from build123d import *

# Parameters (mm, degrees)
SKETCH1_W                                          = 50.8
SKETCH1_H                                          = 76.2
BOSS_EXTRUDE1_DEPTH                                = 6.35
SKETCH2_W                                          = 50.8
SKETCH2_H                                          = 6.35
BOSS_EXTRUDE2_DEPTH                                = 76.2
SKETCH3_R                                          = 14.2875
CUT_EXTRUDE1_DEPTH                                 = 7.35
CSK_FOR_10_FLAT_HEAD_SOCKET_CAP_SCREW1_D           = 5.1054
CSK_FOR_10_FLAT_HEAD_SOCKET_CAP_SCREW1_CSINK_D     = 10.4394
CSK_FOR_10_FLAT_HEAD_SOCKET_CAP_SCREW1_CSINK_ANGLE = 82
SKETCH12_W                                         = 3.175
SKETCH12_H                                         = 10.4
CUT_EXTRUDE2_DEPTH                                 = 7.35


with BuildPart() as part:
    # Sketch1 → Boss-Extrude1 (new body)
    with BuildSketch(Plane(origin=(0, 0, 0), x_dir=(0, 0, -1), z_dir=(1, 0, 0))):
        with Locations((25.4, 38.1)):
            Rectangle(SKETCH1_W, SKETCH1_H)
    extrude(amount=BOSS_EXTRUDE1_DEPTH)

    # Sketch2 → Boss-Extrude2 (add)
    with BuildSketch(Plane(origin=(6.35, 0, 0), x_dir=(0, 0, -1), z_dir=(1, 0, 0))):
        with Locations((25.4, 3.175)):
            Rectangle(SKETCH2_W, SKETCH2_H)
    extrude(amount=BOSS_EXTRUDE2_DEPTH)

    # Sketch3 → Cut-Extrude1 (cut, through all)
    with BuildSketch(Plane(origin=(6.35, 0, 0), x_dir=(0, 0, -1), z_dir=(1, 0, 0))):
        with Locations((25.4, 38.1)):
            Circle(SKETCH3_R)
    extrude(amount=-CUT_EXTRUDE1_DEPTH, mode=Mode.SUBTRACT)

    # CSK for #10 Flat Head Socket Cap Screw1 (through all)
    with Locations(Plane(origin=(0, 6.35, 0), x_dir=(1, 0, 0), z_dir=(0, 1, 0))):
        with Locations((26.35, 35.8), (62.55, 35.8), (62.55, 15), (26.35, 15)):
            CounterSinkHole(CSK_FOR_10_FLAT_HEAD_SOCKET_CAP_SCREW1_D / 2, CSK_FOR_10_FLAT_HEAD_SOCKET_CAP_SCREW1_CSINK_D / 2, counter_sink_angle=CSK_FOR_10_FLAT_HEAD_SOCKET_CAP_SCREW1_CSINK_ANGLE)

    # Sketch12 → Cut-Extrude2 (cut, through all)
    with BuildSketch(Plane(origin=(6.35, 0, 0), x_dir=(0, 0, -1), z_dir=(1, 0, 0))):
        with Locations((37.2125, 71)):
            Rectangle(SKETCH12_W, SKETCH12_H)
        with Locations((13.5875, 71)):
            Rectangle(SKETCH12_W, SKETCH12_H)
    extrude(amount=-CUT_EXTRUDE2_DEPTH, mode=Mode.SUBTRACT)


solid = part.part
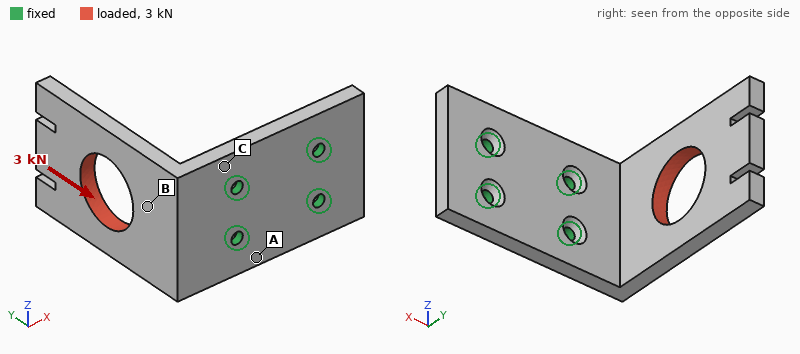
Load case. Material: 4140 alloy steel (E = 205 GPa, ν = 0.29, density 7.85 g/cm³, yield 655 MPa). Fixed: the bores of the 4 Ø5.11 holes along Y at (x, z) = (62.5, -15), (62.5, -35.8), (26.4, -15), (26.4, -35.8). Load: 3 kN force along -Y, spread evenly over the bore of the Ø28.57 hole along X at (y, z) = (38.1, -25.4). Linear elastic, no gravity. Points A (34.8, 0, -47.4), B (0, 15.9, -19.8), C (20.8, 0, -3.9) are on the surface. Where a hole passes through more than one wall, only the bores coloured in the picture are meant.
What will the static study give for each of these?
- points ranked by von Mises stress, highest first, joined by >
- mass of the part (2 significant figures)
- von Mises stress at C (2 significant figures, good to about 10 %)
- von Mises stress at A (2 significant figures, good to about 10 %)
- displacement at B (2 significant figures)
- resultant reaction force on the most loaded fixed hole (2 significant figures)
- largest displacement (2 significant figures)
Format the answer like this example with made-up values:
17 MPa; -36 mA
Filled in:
C > A > B; 340 g; 130 MPa; 54 MPa; 0.12 mm; 2.4 kN; 0.38 mm
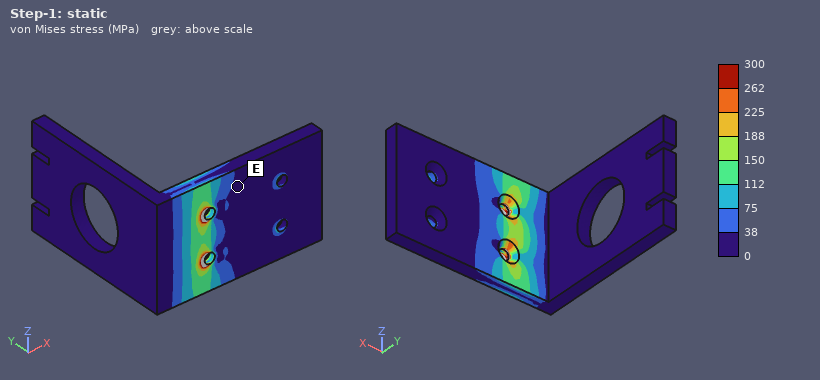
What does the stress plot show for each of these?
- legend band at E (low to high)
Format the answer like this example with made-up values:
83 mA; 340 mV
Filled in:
0 to 38 MPa
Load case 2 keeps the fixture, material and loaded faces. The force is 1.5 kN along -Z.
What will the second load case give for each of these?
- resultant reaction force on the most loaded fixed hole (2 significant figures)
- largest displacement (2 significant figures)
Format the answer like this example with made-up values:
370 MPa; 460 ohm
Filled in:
2.8 kN; 0.19 mm
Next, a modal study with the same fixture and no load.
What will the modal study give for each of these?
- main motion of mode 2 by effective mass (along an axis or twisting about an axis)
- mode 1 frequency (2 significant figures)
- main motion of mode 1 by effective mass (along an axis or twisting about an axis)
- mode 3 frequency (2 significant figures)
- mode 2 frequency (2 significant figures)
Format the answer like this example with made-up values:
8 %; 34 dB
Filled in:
along Z; 640 Hz; along X; 2500 Hz; 1300 Hz
